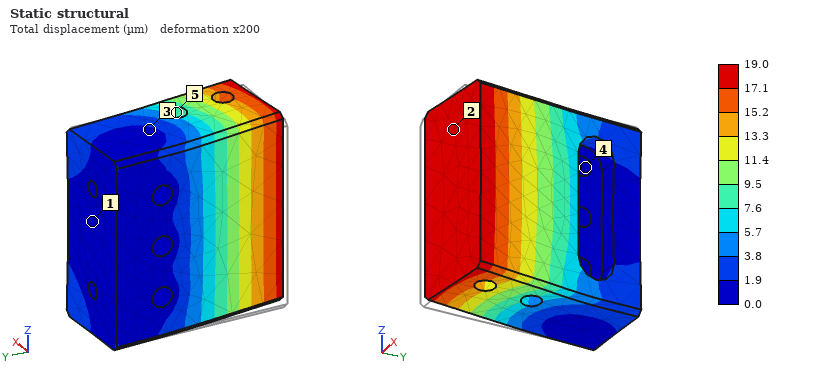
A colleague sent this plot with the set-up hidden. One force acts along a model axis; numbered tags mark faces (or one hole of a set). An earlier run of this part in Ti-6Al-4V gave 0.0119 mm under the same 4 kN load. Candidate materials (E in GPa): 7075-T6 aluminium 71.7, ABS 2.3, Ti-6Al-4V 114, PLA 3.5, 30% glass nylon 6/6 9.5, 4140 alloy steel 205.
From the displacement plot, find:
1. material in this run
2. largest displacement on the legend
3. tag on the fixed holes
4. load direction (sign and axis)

7075-T6 aluminium
19.0 µm
4
+X
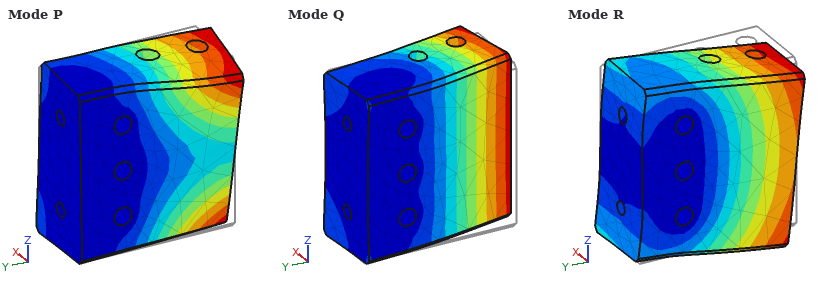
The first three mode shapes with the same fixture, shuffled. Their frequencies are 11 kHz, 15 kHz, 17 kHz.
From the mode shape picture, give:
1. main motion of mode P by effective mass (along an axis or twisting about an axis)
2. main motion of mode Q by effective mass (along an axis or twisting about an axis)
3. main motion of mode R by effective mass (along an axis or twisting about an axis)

twisting about Y
along X
along Z
